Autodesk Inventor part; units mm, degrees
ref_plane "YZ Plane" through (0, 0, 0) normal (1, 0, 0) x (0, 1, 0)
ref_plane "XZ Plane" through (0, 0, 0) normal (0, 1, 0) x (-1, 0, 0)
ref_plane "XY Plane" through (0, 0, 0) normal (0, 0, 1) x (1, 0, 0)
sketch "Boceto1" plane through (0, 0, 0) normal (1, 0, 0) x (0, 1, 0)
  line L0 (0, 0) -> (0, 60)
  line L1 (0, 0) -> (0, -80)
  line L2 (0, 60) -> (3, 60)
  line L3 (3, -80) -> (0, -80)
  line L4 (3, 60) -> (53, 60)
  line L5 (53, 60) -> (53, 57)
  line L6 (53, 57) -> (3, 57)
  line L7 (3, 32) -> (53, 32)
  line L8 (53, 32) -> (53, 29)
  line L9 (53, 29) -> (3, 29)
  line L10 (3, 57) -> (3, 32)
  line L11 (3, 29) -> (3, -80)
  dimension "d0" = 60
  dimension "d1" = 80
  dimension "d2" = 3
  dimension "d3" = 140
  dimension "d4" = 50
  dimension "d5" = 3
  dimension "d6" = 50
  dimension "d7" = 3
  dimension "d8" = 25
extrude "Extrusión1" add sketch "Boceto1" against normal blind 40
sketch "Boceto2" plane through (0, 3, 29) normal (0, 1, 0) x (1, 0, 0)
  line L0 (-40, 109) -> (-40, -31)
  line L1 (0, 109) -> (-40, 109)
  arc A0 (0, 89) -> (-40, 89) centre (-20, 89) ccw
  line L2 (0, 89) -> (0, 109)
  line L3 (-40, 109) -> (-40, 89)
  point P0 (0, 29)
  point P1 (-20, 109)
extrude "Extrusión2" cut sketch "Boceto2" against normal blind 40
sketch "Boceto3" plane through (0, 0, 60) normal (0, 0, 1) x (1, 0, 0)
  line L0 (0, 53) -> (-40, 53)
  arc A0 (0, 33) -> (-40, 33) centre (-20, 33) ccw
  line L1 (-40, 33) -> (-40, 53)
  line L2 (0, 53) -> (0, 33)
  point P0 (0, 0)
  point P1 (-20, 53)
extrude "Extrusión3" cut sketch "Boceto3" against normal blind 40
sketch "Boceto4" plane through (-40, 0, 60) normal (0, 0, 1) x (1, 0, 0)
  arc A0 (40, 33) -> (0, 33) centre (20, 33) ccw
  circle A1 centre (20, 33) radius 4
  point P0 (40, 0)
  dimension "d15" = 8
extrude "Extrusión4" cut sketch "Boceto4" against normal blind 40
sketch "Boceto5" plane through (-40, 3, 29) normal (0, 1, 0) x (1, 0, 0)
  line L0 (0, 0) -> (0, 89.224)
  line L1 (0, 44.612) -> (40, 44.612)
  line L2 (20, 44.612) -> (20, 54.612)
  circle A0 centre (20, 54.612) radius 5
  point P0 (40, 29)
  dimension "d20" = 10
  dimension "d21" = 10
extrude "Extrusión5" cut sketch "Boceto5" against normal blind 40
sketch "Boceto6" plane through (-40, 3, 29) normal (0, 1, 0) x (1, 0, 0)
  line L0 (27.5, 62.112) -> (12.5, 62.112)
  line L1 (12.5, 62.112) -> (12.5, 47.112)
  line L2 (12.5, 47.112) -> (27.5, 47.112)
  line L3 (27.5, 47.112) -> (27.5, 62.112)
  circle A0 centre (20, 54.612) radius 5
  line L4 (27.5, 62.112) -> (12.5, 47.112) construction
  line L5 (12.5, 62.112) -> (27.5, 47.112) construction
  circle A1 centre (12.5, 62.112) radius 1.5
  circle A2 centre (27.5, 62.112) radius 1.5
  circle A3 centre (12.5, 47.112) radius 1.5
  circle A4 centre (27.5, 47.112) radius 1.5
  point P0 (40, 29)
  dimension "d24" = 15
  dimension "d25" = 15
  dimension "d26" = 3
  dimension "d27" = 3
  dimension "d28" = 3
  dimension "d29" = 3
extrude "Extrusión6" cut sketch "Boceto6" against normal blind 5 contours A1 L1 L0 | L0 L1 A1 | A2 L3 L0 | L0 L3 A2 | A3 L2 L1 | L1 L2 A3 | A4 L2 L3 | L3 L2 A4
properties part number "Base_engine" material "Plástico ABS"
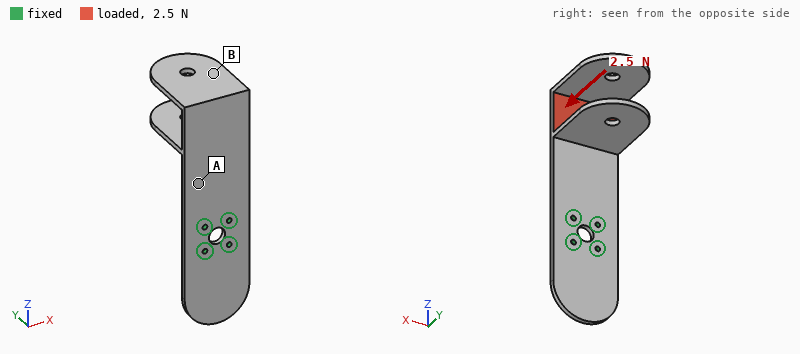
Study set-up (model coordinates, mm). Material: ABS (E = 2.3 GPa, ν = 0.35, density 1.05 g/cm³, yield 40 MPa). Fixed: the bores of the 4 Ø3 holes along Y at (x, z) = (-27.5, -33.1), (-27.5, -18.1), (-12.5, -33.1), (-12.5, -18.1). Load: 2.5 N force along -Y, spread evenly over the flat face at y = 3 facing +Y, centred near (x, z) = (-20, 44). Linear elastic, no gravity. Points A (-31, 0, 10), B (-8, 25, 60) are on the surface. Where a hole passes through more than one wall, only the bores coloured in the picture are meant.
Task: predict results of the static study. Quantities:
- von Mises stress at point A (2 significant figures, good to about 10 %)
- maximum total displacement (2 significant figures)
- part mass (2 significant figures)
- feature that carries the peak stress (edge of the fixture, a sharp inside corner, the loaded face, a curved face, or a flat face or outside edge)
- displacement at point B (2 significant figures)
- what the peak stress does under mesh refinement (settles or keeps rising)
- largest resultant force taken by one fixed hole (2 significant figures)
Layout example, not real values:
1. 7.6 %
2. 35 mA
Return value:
1. 1.4 MPa
2. 1.8 mm
3. 28 g
4. edge of the fixture
5. 1.4 mm
6. keeps rising
7. 2.7 N
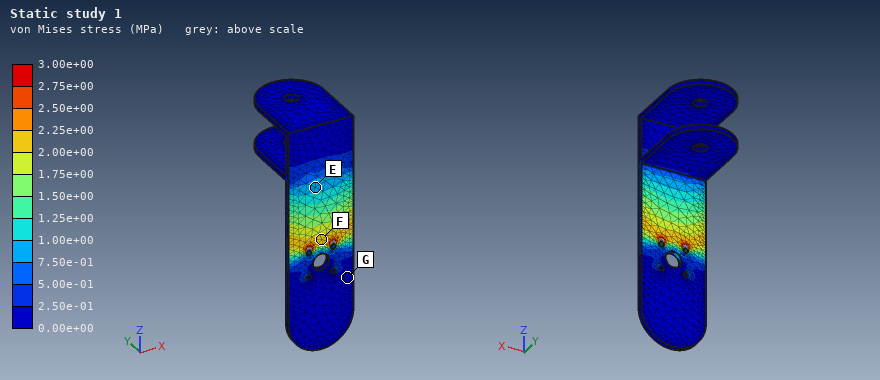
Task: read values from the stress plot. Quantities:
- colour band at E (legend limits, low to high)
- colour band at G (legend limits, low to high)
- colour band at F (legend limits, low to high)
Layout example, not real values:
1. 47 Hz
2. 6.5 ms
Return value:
1. 7.50e-01 to 1.00e+00 MPa
2. 0.00e+00 to 2.50e-01 MPa
3. 2.00e+00 to 2.25e+00 MPa
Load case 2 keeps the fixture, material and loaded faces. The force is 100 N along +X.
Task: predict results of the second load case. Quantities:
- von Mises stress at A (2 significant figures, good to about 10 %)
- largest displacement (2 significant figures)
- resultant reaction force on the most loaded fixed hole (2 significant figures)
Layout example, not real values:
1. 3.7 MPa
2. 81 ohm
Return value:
1. 2.4 MPa
2. 1.7 mm
3. 220 N
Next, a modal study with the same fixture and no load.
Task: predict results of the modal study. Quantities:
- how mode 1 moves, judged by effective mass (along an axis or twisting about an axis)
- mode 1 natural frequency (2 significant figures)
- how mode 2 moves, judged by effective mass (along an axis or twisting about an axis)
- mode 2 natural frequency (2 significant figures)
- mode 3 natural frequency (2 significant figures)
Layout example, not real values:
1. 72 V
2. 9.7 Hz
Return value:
1. along Y
2. 54 Hz
3. along X
4. 130 Hz
5. 200 Hz
